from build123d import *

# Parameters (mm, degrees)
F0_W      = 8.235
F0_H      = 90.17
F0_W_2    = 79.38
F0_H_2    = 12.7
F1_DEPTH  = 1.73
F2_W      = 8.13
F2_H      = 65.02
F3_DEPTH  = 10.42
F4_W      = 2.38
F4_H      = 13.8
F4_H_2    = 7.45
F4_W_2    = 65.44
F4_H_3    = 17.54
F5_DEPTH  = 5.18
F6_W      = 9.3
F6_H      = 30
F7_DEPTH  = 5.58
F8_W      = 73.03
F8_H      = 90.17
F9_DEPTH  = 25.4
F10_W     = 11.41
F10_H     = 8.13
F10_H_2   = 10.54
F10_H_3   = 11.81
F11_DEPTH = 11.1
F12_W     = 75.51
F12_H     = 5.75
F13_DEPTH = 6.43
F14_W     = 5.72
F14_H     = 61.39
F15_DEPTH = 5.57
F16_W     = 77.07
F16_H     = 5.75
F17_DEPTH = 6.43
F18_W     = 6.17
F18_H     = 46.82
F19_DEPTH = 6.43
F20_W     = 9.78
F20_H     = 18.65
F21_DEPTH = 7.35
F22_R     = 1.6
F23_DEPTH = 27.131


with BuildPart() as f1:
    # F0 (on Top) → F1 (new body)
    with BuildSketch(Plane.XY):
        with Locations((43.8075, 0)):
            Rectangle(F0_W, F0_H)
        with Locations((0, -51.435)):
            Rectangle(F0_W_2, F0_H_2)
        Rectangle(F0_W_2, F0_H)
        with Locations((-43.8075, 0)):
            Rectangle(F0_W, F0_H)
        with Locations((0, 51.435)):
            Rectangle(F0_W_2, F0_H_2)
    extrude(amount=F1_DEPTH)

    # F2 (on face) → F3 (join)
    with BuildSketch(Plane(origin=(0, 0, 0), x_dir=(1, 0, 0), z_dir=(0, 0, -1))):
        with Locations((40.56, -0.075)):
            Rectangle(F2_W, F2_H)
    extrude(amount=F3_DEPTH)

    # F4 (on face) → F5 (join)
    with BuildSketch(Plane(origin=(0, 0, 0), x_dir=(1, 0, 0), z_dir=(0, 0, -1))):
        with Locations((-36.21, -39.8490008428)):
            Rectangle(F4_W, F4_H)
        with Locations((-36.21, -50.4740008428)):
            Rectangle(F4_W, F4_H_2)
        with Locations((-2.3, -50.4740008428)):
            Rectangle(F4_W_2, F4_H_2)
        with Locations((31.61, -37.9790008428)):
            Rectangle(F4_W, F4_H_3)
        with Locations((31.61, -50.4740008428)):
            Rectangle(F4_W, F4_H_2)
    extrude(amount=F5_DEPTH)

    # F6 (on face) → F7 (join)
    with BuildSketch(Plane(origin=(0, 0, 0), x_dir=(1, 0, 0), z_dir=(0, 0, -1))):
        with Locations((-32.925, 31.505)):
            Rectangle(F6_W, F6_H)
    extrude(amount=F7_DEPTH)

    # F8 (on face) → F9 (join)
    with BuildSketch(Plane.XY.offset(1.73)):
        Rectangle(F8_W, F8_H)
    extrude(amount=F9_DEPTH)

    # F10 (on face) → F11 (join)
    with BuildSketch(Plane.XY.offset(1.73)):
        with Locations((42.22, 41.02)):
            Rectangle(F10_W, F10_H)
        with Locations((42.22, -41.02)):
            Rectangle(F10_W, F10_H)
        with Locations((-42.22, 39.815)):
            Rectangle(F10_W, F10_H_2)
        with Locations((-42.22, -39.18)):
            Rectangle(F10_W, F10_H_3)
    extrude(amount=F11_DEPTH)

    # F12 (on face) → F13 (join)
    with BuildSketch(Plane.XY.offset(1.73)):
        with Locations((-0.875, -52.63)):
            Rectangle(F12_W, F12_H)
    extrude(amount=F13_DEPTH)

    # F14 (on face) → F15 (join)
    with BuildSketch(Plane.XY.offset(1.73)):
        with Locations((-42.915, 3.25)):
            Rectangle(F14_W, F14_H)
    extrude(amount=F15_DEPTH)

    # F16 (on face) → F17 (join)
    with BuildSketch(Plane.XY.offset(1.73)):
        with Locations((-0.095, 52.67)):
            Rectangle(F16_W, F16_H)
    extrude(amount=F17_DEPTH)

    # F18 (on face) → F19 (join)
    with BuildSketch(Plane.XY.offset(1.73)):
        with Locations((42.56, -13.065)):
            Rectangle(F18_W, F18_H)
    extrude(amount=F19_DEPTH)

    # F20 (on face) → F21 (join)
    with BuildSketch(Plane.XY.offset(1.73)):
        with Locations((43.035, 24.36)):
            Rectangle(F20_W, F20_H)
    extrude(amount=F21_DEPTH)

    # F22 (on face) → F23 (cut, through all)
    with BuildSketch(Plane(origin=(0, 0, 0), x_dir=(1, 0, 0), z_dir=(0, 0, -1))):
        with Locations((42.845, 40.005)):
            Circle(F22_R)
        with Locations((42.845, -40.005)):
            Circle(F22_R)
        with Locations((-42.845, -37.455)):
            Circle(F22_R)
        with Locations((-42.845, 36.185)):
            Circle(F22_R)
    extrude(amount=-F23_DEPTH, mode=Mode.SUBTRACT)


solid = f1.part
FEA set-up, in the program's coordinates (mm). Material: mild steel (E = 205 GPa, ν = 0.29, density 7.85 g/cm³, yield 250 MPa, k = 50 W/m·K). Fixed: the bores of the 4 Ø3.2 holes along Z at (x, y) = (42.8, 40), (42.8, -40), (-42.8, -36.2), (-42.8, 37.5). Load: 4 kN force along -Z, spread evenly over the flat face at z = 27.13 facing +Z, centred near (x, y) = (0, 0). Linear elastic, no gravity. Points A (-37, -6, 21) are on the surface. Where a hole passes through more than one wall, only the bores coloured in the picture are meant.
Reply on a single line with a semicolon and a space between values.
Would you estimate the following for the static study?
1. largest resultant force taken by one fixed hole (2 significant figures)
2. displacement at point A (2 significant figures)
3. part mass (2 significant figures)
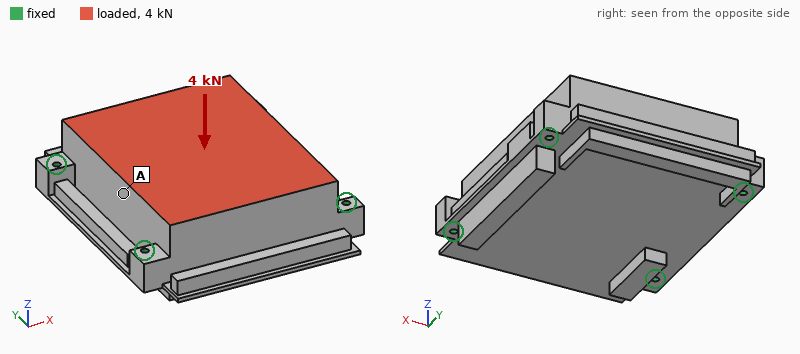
1.1 kN; 2.4 µm; 1.7 kg
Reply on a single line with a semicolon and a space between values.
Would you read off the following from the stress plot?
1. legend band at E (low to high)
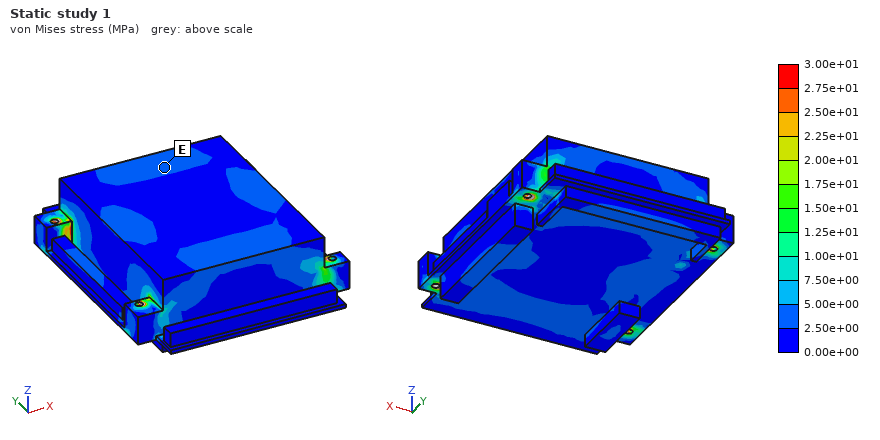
2.50e+00 to 5.00e+00 MPa
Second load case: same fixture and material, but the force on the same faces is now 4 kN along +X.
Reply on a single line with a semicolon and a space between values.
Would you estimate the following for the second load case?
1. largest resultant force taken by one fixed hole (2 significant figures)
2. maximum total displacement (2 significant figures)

1.2 kN; 1.9 µm
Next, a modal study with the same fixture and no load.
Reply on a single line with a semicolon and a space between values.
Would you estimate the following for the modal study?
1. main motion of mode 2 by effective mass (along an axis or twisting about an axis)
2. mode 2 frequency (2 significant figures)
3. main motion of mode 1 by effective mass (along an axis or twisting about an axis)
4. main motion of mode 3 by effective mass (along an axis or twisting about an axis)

along Z; 5300 Hz; along Z; along Y
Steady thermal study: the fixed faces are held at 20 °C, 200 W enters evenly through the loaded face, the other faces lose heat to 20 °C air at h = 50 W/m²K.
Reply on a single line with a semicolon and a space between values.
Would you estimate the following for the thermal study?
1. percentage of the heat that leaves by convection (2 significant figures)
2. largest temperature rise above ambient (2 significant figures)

36 %; 74 K
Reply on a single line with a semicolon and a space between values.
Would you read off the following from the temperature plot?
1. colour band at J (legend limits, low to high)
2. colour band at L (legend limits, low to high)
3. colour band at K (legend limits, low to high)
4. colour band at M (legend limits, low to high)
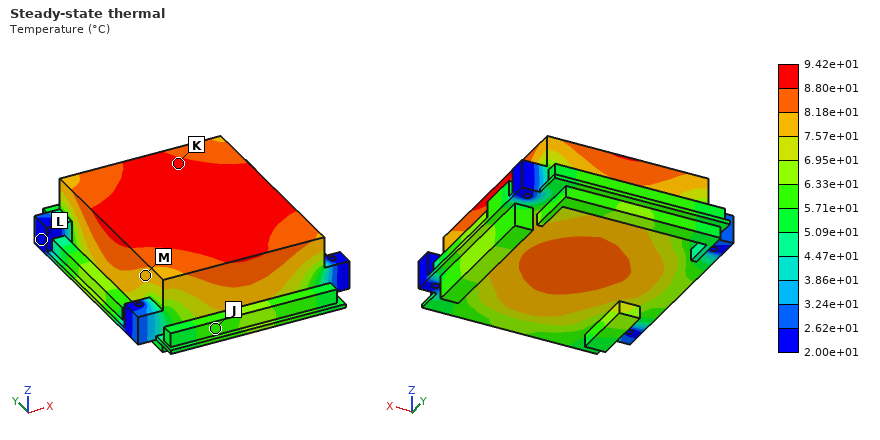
5.71e+01 to 6.33e+01 °C; 2.00e+01 to 2.62e+01 °C; 8.80e+01 to 9.42e+01 °C; 7.57e+01 to 8.18e+01 °C
